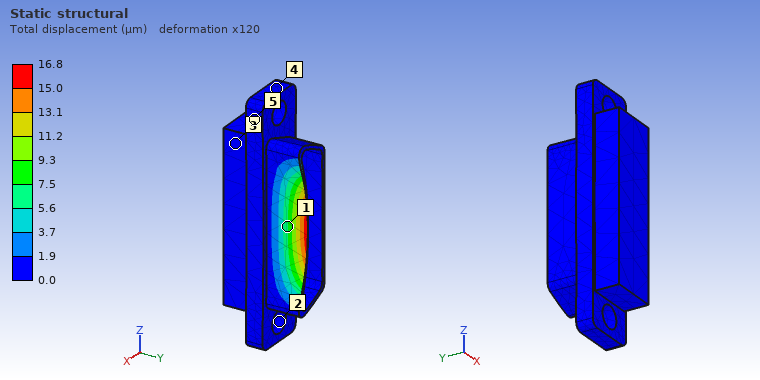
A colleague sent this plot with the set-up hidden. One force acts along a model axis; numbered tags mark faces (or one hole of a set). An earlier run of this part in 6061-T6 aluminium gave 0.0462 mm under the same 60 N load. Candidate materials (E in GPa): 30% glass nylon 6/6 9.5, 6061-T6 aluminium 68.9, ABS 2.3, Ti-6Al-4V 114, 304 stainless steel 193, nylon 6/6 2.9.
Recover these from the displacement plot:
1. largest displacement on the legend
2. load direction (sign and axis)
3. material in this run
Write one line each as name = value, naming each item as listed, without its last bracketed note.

largest displacement on the legend = 16.8 µm
load direction = -X
material in this run = 304 stainless steel
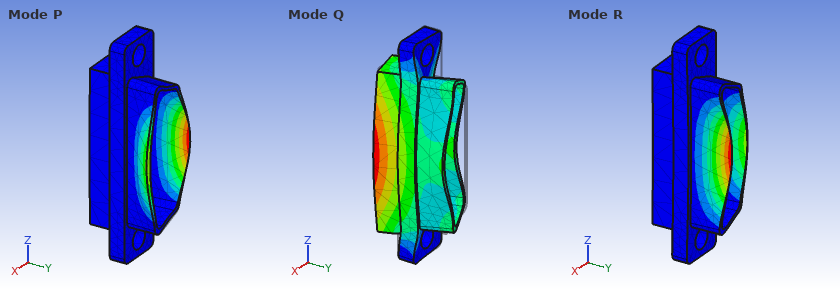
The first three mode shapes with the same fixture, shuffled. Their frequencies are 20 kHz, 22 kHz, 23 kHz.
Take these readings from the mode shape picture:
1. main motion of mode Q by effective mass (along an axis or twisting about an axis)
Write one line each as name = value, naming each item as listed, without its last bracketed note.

main motion of mode Q by effective mass = along X
